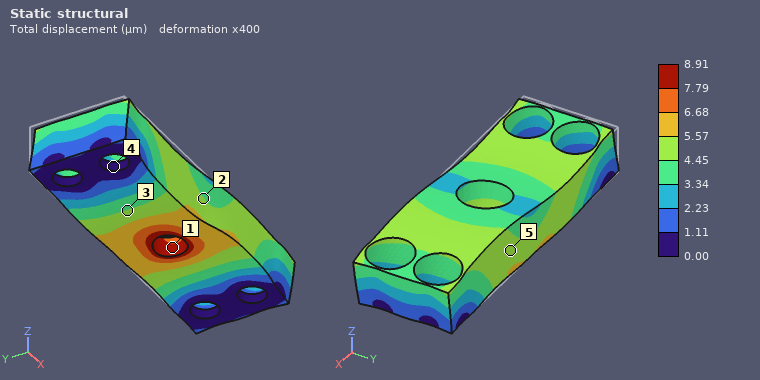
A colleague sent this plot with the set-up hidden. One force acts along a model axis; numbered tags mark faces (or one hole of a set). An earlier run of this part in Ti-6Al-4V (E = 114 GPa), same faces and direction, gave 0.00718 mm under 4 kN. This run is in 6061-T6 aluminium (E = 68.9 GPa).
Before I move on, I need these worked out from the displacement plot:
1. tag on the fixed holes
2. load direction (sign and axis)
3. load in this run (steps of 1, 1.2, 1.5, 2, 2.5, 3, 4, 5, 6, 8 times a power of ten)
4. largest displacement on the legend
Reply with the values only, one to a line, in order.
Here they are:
4
+X
3 kN
8.91 µm
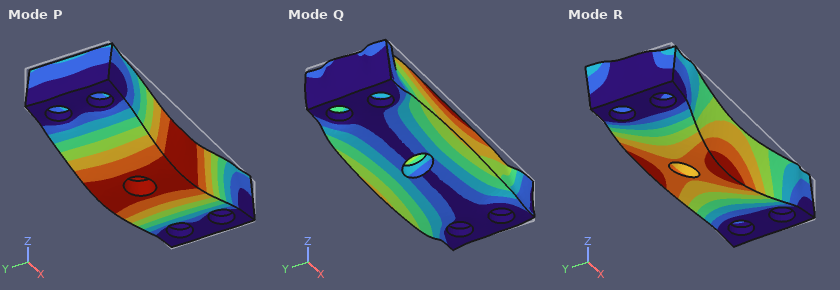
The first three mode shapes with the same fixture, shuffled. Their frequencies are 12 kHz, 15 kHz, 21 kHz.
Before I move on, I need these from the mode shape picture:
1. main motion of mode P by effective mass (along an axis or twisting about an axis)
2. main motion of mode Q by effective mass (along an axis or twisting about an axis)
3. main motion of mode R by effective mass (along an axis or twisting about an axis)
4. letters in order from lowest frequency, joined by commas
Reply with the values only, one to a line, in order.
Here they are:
along Z
along Y
along Y
P, Q, R
